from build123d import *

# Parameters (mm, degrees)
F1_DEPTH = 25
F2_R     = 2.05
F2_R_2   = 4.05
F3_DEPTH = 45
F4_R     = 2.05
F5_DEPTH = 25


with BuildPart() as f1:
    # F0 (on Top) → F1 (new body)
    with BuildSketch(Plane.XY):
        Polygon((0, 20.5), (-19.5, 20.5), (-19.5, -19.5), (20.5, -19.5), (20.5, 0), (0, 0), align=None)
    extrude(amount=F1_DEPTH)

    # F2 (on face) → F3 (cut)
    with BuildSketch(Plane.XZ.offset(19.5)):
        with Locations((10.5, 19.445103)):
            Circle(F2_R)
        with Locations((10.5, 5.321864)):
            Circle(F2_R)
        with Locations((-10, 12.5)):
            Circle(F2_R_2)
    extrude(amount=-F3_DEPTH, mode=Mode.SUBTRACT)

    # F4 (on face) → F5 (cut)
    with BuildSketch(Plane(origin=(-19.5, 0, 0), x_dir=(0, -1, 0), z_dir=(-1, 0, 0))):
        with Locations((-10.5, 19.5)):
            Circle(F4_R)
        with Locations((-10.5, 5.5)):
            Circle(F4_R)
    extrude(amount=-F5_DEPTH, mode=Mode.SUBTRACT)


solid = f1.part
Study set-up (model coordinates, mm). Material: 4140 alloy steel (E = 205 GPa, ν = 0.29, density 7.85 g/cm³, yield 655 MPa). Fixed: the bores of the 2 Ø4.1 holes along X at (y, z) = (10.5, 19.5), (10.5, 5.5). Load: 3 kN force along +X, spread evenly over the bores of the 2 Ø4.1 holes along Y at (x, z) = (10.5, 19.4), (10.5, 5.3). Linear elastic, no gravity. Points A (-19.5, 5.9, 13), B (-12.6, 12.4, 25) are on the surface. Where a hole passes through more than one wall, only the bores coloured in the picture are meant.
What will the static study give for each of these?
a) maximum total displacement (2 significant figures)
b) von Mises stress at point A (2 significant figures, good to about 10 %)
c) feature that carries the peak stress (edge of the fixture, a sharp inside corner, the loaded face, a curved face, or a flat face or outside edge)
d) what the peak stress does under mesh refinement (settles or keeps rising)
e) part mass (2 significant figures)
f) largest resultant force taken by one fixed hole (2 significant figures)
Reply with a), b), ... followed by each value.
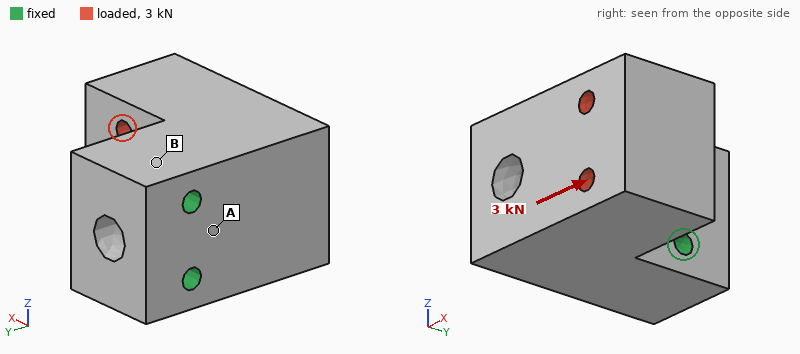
a) 11 µm
b) 20 MPa
c) edge of the fixture
d) keeps rising
e) 210 g
f) 1.5 kN
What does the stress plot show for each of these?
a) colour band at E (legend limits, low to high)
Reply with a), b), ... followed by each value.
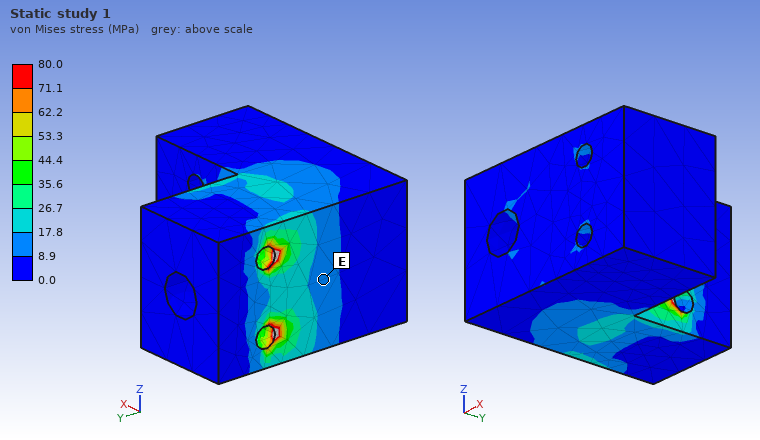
a) 8.9 to 17.8 MPa
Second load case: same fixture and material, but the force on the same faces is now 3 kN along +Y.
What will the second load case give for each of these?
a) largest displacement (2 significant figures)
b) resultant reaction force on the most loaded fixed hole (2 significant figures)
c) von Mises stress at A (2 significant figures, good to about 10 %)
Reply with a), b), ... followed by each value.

a) 17 µm
b) 1.5 kN
c) 22 MPa
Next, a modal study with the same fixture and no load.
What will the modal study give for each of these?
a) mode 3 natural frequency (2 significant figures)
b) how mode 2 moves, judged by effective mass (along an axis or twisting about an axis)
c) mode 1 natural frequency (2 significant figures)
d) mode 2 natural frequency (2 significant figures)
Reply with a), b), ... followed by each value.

a) 15 kHz
b) along Z
c) 7600 Hz
d) 8500 Hz
